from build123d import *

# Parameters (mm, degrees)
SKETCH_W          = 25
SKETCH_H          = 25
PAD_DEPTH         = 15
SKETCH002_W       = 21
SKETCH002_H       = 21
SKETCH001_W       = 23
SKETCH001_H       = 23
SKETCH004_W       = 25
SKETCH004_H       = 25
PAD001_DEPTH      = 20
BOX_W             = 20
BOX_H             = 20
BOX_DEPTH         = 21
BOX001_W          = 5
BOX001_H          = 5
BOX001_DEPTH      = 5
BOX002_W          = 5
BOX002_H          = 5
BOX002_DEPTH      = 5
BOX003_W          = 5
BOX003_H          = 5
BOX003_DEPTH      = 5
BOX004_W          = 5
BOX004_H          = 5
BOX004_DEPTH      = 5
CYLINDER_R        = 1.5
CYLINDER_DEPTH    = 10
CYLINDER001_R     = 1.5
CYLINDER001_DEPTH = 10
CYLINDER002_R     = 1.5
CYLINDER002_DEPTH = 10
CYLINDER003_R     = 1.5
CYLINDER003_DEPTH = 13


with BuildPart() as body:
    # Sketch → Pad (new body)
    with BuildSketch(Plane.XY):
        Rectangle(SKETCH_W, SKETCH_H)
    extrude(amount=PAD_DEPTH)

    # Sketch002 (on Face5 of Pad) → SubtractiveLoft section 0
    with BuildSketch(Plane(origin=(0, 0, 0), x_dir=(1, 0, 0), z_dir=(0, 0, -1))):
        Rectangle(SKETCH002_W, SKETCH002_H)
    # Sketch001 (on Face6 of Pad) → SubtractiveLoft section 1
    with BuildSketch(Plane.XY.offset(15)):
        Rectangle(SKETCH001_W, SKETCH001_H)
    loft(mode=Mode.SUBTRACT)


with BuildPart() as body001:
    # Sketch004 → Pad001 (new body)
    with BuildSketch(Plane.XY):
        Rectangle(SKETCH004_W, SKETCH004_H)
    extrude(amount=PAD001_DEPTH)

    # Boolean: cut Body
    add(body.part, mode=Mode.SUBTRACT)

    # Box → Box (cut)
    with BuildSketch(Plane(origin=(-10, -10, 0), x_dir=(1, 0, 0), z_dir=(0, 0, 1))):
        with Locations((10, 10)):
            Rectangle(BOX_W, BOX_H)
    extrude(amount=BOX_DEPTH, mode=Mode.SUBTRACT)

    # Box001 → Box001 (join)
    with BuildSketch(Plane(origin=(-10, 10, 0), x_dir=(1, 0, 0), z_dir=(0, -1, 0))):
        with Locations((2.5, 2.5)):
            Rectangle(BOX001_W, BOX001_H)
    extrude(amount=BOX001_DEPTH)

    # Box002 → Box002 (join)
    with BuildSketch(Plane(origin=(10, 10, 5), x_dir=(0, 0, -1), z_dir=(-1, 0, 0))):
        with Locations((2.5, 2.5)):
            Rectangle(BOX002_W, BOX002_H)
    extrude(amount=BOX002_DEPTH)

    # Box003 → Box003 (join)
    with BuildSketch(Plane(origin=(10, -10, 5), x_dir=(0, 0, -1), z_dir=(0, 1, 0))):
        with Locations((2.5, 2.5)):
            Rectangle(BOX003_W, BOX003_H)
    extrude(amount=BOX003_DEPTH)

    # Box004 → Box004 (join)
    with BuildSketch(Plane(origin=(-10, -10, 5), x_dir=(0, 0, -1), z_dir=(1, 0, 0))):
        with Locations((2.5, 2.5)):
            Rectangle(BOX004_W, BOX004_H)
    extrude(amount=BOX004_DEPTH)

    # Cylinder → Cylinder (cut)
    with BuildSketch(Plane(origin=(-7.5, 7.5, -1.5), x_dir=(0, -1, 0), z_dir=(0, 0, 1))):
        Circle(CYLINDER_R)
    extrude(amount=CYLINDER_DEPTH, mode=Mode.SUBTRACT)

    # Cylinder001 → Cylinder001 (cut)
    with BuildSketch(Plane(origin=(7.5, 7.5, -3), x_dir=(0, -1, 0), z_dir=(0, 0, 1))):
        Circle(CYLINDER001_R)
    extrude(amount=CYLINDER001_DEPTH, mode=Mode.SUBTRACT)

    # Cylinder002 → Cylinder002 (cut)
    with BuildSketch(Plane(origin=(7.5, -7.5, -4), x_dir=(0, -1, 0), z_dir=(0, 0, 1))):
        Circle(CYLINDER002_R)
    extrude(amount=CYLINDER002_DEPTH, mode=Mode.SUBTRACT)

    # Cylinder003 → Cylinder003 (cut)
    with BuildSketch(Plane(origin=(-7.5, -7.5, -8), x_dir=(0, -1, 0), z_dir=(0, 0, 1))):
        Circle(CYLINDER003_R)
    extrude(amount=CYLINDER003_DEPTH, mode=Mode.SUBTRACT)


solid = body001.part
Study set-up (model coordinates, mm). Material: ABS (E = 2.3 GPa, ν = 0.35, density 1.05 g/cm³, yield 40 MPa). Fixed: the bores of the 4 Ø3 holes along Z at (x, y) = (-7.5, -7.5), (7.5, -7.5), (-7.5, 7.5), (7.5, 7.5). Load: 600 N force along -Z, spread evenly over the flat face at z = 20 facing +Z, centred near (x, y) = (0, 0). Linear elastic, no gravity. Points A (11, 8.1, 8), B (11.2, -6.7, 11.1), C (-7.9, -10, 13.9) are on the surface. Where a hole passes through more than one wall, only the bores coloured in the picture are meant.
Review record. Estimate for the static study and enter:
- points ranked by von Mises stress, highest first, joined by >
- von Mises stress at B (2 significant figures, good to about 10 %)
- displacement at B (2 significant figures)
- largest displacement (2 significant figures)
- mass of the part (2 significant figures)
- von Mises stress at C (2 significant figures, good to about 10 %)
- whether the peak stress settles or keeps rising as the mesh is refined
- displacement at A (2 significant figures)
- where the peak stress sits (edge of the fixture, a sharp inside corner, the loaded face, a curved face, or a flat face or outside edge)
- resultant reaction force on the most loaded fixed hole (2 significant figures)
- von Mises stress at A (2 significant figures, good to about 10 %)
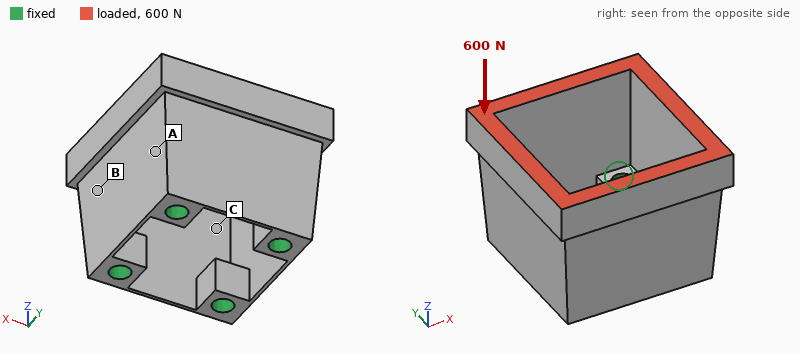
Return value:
A > B > C
6.8 MPa
39 µm
70 µm
2.9 g
3.4 MPa
keeps rising
30 µm
edge of the fixture
150 N
9.0 MPa
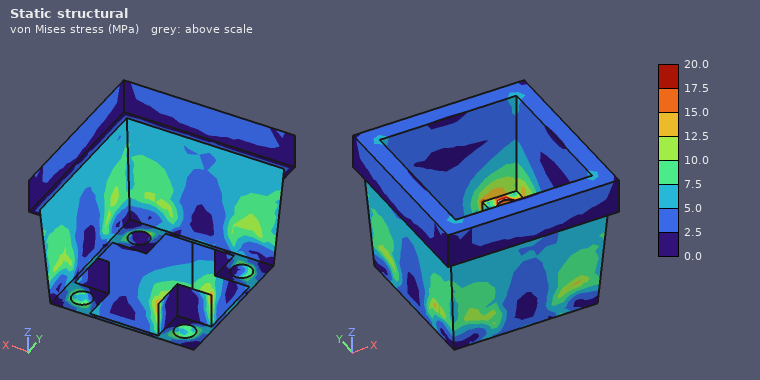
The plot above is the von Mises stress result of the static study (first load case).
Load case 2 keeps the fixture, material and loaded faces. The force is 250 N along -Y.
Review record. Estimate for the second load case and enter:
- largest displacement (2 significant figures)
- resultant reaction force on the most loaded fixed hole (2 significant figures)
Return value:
0.44 mm
130 N
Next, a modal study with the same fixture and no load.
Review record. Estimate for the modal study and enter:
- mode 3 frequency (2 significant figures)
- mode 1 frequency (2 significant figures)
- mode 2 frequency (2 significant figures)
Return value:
4300 Hz
3500 Hz
4300 Hz
